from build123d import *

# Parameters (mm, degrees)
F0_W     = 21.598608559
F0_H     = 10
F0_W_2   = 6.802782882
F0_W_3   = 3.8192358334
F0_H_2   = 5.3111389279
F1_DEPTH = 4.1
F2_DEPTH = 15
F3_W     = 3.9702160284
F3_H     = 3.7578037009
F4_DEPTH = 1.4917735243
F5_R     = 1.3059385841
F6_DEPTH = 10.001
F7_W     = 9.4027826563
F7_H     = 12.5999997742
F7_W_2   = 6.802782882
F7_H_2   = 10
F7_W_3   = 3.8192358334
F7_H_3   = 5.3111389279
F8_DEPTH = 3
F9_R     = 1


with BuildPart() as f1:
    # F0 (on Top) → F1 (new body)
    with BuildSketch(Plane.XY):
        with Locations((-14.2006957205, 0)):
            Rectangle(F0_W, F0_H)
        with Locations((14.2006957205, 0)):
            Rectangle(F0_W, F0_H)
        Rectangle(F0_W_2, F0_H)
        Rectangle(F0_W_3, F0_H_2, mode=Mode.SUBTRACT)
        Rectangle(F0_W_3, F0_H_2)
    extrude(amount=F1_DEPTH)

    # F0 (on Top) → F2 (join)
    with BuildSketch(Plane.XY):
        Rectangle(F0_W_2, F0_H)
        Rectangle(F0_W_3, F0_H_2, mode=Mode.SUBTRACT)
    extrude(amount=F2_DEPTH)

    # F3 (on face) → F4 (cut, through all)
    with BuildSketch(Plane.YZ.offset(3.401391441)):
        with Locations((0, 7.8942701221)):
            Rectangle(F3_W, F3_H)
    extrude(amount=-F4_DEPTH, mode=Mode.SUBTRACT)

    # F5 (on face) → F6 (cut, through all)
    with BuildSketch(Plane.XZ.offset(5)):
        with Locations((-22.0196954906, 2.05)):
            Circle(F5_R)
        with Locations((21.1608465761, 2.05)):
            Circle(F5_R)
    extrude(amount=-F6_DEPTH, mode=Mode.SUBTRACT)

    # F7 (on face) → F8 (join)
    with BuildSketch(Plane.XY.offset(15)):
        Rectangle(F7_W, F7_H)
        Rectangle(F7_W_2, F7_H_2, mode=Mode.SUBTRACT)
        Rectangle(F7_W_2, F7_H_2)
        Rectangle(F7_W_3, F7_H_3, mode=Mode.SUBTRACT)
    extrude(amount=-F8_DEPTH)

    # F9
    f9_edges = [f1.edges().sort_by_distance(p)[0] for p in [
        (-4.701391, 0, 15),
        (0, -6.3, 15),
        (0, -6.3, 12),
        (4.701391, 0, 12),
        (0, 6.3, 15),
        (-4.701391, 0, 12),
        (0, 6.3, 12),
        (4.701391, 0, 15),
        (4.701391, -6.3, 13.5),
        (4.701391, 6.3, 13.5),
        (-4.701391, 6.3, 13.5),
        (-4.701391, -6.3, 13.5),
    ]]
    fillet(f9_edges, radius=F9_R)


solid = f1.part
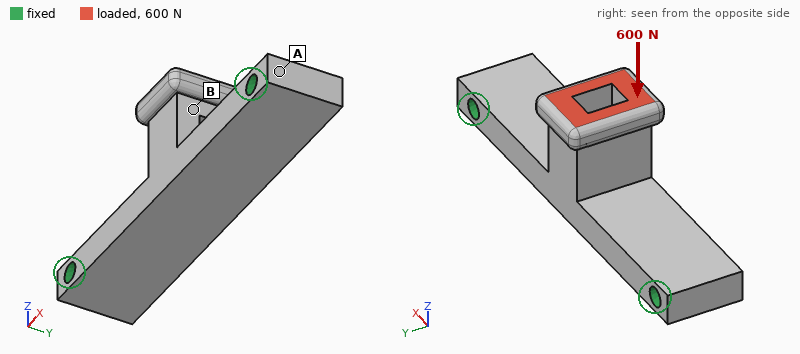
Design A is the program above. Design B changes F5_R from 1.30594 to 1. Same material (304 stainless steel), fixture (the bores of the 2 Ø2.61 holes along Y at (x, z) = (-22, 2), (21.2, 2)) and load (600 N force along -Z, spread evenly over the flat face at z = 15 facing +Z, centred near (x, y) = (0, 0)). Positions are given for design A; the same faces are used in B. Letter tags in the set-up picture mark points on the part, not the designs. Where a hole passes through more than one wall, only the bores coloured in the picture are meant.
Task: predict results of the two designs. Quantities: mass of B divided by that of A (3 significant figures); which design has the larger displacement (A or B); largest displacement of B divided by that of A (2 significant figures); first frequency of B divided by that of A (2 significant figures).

1.02
B
1.1
0.99
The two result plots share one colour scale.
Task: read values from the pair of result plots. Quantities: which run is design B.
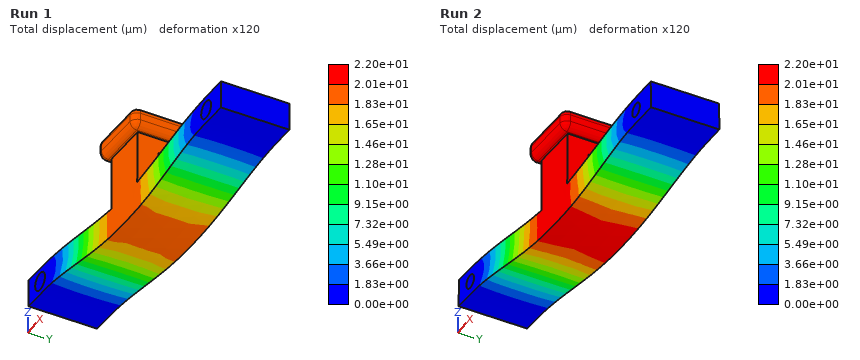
Run 2
